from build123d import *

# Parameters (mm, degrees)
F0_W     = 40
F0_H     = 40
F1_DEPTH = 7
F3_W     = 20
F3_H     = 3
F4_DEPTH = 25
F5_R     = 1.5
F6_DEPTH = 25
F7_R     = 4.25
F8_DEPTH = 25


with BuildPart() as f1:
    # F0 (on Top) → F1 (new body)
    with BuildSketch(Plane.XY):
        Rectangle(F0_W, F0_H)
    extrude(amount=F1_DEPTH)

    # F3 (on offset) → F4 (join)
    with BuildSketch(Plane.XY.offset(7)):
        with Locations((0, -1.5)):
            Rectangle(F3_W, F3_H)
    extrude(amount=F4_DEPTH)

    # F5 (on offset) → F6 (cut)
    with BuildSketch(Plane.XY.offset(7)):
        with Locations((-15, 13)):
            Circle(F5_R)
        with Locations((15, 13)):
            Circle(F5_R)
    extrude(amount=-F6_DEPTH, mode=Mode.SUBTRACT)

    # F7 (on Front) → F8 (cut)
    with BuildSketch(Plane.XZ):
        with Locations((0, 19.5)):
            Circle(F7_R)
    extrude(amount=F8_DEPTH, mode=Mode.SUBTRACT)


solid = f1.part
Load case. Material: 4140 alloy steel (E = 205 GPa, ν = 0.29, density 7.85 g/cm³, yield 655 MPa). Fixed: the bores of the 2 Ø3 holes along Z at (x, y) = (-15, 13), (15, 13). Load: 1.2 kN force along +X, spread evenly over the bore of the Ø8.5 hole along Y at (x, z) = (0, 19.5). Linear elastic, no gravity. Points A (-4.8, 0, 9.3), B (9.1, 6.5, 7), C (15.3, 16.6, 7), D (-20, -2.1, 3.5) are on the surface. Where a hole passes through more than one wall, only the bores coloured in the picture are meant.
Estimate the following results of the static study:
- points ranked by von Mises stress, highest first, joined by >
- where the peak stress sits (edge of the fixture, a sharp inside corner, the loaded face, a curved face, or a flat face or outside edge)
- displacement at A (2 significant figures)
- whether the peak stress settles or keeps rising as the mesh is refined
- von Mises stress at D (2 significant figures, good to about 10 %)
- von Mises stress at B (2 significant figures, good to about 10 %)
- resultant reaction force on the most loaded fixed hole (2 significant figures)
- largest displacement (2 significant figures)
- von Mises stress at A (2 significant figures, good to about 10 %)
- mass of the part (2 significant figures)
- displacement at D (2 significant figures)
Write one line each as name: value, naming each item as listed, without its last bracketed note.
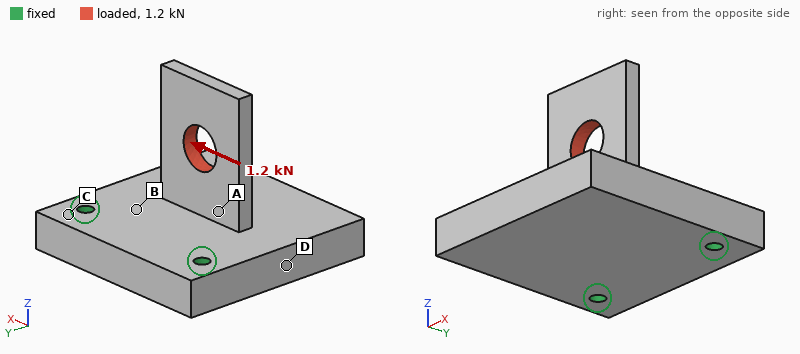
points ranked by von Mises stress, highest first, joined by >: A > B > D > C
where the peak stress sits: edge of the fixture
displacement at A: 5.0 µm
whether the peak stress settles or keeps rising as the mesh is refined: keeps rising
von Mises stress at D: 17 MPa
von Mises stress at B: 30 MPa
resultant reaction force on the most loaded fixed hole: 1.0 kN
largest displacement: 27 µm
von Mises stress at A: 44 MPa
mass of the part: 98 g
displacement at D: 5.9 µm
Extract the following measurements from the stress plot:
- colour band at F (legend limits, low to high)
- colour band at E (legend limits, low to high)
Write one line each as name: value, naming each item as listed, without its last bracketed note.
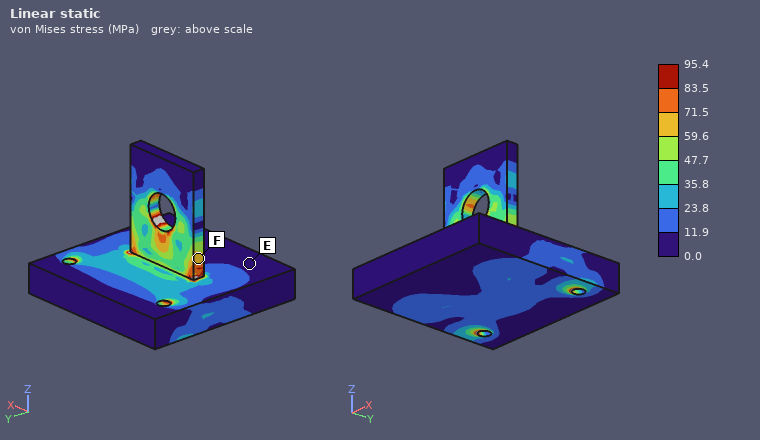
colour band at F: 59.6 to 71.5 MPa
colour band at E: 0.0 to 11.9 MPa
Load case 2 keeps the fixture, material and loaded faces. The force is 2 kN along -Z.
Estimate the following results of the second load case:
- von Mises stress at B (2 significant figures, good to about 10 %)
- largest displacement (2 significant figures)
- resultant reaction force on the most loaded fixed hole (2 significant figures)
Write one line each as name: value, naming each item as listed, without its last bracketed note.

von Mises stress at B: 44 MPa
largest displacement: 45 µm
resultant reaction force on the most loaded fixed hole: 1.0 kN
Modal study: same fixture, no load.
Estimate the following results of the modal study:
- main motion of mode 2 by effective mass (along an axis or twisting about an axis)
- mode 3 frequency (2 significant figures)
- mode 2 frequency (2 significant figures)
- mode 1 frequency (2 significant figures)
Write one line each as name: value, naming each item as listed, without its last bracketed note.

main motion of mode 2 by effective mass: along Z
mode 3 frequency: 8800 Hz
mode 2 frequency: 4700 Hz
mode 1 frequency: 3200 Hz
